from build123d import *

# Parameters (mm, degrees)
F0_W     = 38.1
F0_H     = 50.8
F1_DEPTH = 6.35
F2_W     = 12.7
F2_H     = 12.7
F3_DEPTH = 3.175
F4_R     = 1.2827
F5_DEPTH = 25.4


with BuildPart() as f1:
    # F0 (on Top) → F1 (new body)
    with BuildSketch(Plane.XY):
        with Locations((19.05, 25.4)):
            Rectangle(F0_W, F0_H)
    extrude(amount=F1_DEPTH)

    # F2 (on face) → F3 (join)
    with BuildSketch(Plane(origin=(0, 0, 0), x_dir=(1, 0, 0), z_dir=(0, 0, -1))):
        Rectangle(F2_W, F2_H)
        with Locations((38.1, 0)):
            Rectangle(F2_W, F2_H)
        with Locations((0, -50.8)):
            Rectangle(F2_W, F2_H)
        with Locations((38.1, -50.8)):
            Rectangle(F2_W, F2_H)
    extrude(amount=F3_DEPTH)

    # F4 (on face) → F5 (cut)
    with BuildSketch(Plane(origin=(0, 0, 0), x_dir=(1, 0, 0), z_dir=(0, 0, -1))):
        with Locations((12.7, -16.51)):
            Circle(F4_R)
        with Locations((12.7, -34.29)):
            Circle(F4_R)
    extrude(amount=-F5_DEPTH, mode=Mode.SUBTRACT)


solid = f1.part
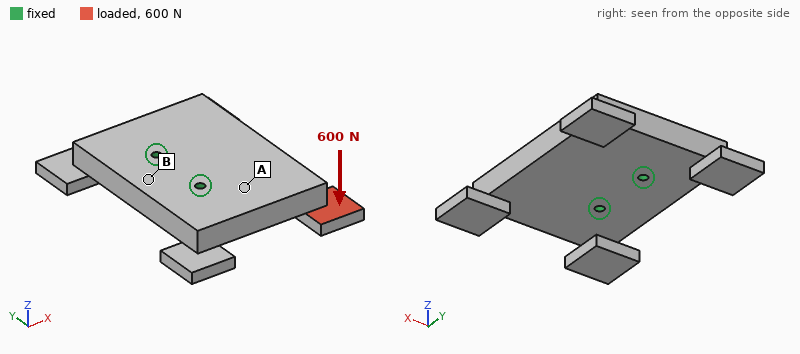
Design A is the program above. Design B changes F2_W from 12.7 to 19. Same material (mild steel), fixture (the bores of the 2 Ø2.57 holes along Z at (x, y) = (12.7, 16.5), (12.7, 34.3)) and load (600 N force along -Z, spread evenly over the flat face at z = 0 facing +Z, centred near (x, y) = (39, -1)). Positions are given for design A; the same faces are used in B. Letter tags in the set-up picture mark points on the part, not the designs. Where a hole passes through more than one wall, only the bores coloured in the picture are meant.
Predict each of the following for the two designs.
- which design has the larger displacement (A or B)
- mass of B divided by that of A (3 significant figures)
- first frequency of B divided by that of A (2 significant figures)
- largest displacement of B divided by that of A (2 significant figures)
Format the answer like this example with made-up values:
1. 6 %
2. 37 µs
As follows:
1. B
2. 1.07
3. 0.91
4. 1.1
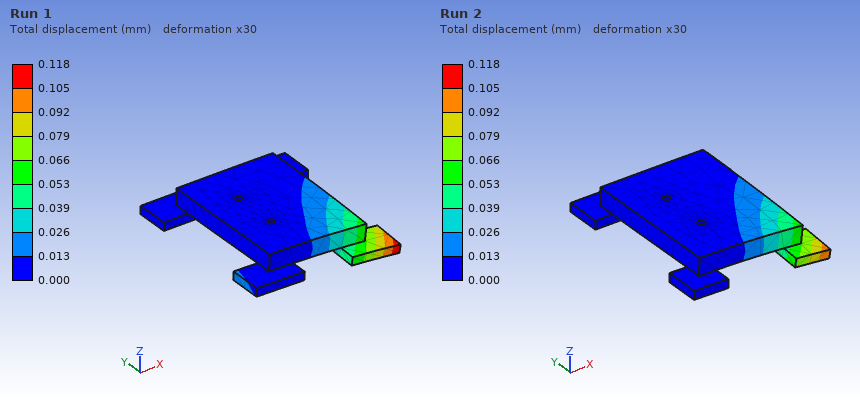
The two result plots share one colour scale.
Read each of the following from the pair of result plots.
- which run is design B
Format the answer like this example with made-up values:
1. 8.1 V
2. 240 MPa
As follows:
1. Run 1
